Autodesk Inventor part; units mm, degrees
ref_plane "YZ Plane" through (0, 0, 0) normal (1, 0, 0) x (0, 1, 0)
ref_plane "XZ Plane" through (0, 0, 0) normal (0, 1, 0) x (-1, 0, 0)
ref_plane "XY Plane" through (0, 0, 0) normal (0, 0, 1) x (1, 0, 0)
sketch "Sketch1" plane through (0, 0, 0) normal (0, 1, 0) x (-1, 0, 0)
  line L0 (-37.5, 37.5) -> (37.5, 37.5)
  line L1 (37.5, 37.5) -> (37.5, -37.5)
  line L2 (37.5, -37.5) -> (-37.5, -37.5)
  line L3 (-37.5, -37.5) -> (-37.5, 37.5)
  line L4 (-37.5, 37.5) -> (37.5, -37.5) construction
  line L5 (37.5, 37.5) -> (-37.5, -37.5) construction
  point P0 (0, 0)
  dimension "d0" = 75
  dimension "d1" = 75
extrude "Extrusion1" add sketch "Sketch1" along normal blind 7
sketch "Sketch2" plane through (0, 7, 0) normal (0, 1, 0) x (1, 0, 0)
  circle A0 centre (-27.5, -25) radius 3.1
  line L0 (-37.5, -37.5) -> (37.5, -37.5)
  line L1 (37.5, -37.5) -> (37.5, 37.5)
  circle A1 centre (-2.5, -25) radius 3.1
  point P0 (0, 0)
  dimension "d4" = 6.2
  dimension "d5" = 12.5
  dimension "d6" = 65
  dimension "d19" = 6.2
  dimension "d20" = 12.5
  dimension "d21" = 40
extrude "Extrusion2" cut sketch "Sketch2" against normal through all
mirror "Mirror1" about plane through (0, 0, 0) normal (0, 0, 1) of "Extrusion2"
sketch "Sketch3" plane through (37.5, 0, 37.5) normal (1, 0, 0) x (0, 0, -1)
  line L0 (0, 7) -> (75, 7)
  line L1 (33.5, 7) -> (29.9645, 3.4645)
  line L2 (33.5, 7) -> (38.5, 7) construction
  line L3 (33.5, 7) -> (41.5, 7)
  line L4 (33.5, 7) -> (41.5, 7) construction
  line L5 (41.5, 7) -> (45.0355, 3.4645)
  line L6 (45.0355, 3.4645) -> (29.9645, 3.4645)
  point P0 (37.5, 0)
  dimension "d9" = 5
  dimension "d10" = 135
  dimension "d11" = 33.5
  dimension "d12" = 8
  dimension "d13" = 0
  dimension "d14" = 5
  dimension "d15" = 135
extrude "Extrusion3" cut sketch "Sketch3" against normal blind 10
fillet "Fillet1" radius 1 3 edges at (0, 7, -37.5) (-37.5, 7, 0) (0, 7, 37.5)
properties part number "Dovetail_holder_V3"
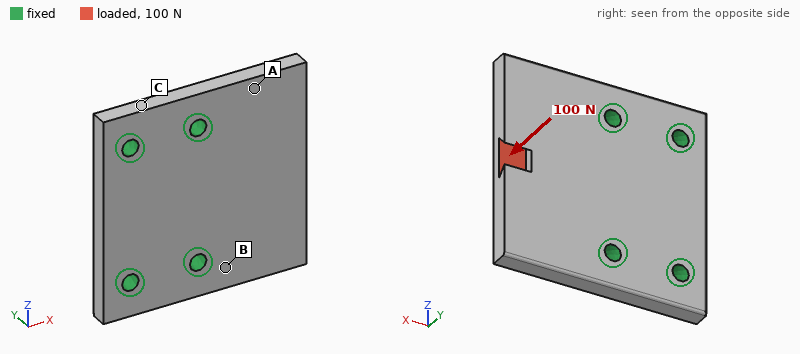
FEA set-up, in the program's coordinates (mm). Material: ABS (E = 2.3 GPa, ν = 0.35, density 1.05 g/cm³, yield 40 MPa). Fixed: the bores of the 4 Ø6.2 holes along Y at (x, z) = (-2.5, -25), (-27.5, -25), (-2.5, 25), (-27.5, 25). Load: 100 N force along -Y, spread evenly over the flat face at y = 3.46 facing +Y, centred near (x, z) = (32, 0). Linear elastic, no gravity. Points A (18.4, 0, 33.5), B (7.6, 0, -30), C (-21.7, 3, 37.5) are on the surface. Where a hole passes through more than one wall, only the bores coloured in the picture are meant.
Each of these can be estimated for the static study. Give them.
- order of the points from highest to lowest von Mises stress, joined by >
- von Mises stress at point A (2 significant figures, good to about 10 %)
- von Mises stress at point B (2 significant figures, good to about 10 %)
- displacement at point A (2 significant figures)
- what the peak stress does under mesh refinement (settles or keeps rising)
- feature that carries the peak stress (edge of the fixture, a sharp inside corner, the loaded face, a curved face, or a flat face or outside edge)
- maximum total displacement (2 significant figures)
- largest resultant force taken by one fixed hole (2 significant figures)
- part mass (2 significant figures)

B > A > C
2.6 MPa
4.3 MPa
0.10 mm
keeps rising
edge of the fixture
0.53 mm
74 N
40 g
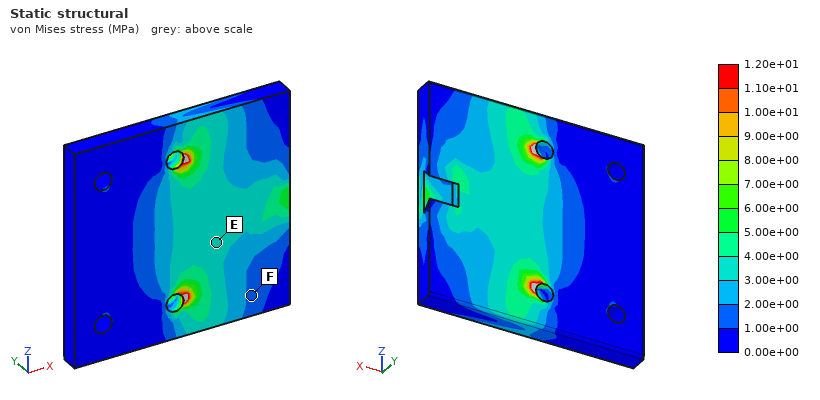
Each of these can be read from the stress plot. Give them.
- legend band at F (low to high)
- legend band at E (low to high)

1.00e+00 to 2.00e+00 MPa
3.00e+00 to 4.00e+00 MPa
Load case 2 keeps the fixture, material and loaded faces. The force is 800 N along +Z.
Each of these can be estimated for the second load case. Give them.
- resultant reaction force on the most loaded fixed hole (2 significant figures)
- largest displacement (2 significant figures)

580 N
0.17 mm
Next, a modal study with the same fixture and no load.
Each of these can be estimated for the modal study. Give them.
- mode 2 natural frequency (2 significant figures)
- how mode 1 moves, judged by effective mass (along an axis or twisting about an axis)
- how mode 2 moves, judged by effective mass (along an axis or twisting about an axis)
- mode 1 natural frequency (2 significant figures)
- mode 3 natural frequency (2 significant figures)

1600 Hz
along Y
twisting about X
1000 Hz
2700 Hz
